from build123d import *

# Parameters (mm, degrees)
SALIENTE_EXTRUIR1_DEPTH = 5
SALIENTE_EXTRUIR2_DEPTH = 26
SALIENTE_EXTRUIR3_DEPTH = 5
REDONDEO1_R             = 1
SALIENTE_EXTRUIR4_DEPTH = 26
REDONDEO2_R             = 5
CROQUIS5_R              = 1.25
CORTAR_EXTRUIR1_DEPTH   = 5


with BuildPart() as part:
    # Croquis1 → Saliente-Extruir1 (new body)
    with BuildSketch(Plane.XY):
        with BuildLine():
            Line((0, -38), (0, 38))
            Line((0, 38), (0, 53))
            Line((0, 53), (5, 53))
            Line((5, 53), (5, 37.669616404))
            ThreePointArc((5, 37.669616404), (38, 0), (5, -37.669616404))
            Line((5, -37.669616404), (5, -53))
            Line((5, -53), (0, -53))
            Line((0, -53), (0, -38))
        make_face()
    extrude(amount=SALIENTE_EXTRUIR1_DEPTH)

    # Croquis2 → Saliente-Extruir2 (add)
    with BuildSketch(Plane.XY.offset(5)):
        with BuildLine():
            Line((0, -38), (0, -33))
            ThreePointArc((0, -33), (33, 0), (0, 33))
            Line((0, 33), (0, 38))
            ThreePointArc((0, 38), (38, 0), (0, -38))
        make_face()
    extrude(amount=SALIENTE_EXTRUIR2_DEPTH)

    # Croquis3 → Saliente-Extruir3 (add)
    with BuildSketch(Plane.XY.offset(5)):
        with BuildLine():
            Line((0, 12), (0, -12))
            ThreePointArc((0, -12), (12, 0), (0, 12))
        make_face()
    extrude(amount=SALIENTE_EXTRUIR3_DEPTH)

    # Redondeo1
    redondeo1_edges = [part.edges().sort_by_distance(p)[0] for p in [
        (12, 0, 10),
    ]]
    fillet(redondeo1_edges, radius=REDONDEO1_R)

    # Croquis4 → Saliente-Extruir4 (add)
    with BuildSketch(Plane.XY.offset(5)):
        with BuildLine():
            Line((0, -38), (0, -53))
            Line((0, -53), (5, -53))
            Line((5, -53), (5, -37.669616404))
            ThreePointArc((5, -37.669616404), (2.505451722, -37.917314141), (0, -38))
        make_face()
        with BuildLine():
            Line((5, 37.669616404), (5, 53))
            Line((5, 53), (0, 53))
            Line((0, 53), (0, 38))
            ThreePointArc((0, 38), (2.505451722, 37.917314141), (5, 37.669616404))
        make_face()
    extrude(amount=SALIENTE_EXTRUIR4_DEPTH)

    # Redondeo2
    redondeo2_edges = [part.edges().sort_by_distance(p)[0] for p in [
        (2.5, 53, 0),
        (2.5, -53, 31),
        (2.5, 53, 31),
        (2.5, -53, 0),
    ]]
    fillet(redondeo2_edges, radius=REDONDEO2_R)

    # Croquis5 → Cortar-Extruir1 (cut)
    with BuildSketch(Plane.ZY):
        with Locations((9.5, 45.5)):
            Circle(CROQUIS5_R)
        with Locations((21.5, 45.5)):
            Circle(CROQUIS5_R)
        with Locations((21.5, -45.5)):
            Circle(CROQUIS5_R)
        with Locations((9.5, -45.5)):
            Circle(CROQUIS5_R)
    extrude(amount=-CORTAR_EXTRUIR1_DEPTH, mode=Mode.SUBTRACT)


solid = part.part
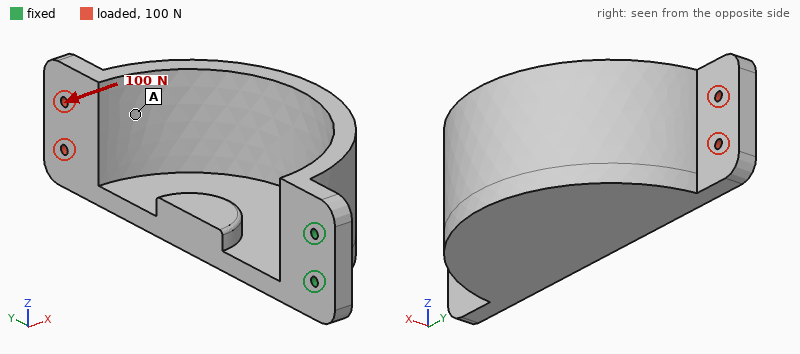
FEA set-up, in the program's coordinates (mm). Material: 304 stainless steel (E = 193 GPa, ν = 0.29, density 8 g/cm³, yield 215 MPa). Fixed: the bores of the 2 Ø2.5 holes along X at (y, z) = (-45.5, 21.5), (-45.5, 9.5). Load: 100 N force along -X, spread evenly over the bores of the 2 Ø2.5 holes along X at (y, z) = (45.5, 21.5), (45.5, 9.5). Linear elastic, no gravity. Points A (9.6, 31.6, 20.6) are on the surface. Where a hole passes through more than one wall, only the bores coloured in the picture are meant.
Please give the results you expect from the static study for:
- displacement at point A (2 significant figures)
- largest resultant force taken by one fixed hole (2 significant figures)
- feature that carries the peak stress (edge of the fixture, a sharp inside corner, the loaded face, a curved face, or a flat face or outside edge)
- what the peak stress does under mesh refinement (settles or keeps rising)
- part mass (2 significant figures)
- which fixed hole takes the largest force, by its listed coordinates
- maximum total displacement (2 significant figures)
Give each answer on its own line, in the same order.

0.17 mm
77 N
edge of the fixture
keeps rising
250 g
(-45.5, 21.5)
0.23 mm
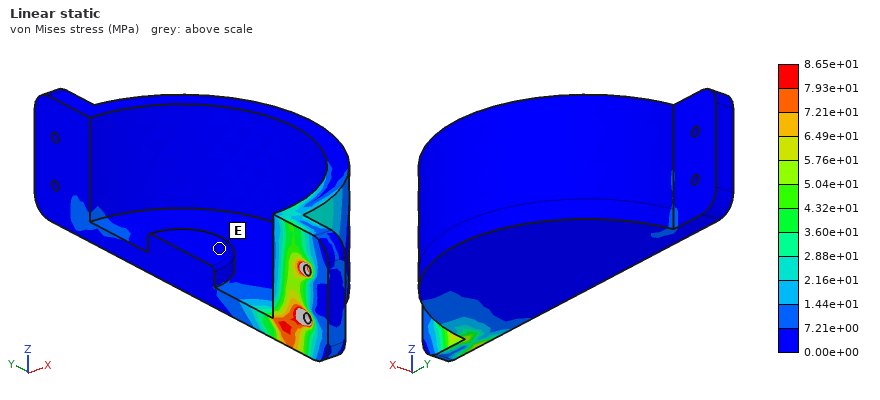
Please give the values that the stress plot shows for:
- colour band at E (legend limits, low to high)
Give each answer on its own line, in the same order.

0.00e+00 to 7.21e+00 MPa
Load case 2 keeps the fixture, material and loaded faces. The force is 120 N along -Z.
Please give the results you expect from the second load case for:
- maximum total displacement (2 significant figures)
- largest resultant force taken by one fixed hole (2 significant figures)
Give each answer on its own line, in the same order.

0.17 mm
800 N
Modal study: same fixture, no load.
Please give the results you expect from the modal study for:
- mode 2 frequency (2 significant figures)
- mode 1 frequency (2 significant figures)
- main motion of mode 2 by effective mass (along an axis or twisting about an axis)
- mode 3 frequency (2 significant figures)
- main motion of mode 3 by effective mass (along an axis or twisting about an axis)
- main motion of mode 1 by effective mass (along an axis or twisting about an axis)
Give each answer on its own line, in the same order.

600 Hz
370 Hz
along Z
2000 Hz
along Z
along X
